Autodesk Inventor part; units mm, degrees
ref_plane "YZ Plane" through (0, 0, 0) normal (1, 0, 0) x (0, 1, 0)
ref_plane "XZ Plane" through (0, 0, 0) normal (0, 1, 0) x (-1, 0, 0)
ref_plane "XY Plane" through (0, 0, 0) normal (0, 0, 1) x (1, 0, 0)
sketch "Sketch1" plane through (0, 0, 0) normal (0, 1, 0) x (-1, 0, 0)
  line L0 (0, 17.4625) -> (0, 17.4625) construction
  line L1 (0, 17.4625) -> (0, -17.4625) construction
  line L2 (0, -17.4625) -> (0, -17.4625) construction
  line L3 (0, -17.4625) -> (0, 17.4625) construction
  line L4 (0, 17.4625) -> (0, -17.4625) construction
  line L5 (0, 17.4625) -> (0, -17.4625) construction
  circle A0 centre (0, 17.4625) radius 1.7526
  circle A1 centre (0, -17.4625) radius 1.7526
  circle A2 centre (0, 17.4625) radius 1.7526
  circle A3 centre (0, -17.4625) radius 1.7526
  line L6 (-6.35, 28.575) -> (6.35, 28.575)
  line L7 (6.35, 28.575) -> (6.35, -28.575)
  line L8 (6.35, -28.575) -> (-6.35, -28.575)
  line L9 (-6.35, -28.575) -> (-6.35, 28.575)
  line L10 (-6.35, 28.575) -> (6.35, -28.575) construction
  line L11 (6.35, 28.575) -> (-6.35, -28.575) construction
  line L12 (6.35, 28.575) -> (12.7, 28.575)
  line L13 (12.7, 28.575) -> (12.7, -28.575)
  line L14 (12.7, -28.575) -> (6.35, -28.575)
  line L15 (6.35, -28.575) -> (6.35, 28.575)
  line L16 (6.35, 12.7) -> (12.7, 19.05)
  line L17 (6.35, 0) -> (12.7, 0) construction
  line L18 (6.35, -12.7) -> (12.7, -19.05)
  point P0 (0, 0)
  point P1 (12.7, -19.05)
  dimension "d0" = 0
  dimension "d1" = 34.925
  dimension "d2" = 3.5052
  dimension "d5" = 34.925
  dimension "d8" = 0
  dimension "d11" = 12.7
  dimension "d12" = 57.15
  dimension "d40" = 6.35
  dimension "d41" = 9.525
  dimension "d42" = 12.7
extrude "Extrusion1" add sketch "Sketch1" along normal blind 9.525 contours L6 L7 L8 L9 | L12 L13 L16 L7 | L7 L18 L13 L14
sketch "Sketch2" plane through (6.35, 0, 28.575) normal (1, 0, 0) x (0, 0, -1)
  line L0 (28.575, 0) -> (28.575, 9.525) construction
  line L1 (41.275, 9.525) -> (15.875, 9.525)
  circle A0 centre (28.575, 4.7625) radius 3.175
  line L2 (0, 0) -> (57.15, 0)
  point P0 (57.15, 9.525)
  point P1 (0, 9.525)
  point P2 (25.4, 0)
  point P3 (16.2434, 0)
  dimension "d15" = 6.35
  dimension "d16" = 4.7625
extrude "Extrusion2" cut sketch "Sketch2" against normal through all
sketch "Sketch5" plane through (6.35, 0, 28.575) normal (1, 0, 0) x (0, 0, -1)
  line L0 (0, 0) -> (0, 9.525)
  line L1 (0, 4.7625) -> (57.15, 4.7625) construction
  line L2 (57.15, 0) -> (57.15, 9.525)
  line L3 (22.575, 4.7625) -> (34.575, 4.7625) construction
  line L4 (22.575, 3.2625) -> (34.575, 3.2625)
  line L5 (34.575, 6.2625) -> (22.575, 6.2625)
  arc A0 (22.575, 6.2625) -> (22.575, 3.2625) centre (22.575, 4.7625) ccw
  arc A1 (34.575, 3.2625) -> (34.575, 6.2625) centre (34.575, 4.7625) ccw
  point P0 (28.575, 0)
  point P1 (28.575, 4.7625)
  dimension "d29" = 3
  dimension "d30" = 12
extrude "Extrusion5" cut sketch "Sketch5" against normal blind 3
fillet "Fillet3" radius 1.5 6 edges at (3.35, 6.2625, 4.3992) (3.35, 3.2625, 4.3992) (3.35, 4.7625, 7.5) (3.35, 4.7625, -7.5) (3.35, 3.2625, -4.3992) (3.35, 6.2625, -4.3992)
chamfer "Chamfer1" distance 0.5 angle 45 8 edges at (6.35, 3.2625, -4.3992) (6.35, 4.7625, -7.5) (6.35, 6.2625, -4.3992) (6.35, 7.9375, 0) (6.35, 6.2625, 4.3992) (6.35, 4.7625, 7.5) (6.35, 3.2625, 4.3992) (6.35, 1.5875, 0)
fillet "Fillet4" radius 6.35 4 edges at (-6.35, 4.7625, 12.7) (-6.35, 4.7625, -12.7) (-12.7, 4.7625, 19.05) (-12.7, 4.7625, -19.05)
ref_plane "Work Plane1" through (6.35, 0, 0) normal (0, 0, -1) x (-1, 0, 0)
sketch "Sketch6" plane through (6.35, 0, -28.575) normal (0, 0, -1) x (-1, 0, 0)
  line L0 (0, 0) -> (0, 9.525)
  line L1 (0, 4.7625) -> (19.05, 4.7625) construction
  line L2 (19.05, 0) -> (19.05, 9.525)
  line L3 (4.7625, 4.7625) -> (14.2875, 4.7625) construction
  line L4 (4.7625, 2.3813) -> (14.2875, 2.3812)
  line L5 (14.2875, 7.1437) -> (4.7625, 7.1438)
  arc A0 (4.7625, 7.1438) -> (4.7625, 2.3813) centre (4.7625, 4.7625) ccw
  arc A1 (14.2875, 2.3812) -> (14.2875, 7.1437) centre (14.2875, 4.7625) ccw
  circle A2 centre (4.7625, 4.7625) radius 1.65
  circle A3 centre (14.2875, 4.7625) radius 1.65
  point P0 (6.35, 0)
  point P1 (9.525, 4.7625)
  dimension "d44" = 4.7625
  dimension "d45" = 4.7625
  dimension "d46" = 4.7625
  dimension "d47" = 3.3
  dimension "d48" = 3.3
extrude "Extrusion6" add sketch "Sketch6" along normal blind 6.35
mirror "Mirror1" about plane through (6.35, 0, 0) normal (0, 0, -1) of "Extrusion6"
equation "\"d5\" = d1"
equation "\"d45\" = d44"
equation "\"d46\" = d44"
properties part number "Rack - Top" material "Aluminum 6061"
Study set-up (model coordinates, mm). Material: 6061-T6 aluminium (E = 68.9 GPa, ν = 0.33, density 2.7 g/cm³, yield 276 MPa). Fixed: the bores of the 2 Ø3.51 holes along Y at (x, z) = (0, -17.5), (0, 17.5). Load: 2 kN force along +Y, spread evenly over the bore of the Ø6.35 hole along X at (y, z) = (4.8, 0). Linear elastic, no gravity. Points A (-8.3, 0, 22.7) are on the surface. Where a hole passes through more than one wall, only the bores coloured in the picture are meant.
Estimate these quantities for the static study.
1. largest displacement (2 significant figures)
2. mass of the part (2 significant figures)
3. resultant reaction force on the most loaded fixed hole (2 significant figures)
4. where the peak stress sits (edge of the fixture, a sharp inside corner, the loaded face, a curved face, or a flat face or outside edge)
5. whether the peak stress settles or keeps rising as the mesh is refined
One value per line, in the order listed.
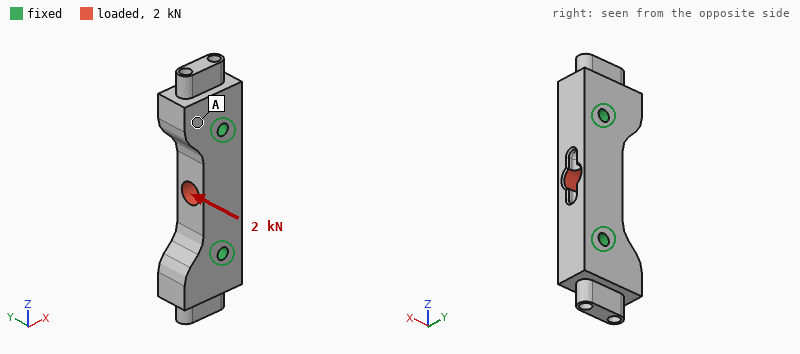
15 µm
23 g
1.0 kN
edge of the fixture
keeps rising
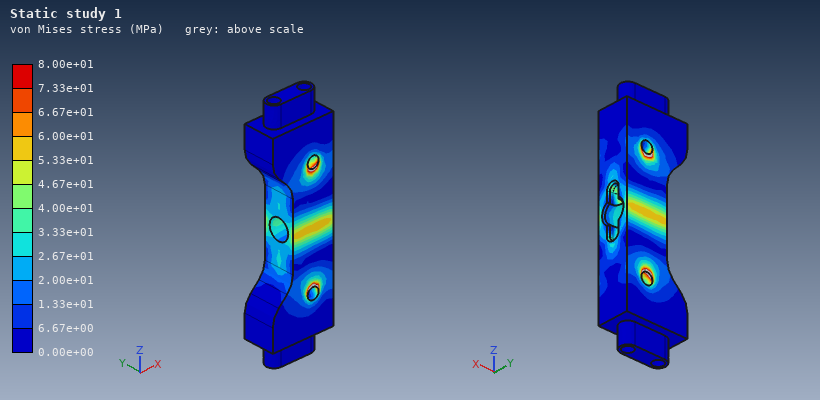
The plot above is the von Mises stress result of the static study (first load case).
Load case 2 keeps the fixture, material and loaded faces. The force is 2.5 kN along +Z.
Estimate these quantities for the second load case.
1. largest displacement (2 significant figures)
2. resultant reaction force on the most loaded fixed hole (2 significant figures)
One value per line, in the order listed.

3.0 µm
1.3 kN
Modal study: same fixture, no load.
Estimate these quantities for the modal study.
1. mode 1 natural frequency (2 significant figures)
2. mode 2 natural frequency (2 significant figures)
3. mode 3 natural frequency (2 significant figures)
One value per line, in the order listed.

18 kHz
24 kHz
24 kHz
